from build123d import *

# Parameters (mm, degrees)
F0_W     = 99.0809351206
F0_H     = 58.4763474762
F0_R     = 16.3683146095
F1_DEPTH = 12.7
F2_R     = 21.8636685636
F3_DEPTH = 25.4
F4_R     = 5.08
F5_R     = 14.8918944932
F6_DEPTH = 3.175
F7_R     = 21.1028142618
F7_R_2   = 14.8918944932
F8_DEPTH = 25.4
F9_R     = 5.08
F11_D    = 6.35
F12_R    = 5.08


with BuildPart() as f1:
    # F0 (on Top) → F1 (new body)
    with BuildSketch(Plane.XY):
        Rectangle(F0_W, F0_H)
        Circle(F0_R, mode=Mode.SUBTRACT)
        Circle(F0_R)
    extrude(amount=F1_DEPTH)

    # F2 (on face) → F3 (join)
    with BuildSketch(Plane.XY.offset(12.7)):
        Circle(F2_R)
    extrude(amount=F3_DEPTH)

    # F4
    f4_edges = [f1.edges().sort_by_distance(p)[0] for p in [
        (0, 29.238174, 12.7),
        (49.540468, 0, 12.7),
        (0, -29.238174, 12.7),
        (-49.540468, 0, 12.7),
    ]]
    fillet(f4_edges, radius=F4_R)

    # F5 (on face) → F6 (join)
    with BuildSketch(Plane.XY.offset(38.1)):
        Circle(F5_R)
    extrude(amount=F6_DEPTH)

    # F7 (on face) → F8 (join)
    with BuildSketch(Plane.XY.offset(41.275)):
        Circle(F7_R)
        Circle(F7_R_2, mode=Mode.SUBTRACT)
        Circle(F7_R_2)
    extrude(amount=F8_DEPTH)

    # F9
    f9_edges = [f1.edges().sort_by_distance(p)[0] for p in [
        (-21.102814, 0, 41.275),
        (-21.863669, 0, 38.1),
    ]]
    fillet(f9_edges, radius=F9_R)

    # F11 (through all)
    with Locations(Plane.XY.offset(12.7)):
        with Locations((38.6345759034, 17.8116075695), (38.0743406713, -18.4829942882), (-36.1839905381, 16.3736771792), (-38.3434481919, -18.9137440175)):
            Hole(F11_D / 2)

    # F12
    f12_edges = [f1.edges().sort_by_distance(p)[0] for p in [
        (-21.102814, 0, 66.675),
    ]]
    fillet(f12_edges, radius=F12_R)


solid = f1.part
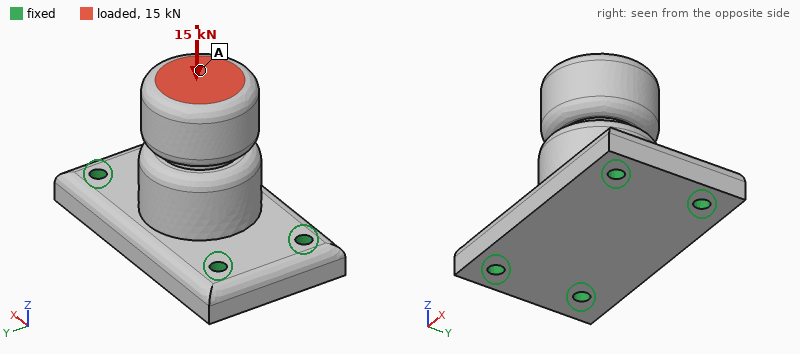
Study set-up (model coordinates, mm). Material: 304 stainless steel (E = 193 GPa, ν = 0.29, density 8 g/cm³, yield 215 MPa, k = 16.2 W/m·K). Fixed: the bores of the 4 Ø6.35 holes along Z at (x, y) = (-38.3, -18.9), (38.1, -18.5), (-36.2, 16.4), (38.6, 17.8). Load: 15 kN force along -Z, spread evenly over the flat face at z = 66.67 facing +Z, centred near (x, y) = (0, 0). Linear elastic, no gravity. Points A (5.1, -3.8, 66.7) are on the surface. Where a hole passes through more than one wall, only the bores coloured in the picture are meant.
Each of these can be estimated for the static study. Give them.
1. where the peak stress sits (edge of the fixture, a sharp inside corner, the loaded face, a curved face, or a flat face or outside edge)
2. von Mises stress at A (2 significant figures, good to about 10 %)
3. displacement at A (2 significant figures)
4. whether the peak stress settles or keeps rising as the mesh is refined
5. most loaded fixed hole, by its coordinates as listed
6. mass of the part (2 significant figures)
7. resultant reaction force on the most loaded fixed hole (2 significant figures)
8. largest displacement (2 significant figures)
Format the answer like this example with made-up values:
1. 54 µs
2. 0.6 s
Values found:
1. edge of the fixture
2. 12 MPa
3. 16 µm
4. keeps rising
5. (-36.2, 16.4)
6. 1.2 kg
7. 4.5 kN
8. 16 µm
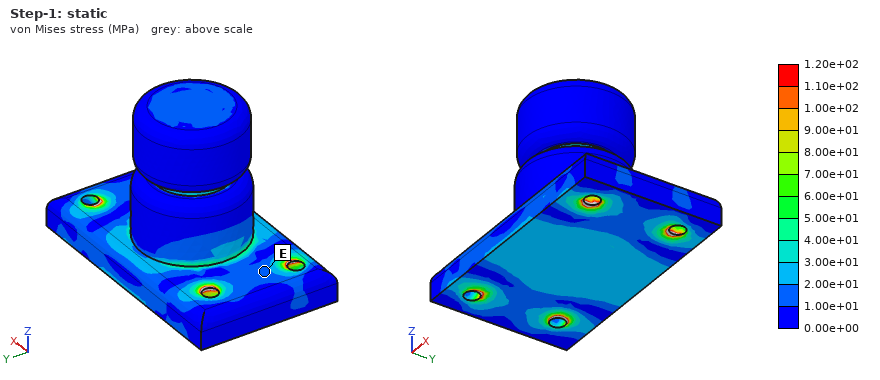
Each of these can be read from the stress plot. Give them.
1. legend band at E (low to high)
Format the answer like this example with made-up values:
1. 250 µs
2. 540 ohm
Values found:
1. 1.00e+01 to 2.00e+01 MPa
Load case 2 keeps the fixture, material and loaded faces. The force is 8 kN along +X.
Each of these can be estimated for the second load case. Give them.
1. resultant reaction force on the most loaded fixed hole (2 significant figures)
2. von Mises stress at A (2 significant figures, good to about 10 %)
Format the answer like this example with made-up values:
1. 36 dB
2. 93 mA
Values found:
1. 5.0 kN
2. 18 MPa
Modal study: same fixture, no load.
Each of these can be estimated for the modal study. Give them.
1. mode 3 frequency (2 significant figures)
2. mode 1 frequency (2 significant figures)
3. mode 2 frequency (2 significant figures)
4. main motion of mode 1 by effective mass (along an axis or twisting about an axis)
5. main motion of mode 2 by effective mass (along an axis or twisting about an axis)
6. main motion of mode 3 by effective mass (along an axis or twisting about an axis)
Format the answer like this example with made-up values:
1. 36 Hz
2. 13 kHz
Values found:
1. 6100 Hz
2. 3200 Hz
3. 4600 Hz
4. along Y
5. along X
6. along Z
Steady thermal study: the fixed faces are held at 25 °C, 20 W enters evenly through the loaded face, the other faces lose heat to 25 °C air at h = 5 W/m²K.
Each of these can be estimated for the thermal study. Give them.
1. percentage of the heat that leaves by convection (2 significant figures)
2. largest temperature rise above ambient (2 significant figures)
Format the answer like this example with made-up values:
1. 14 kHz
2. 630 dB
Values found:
1. 13 %
2. 80 K
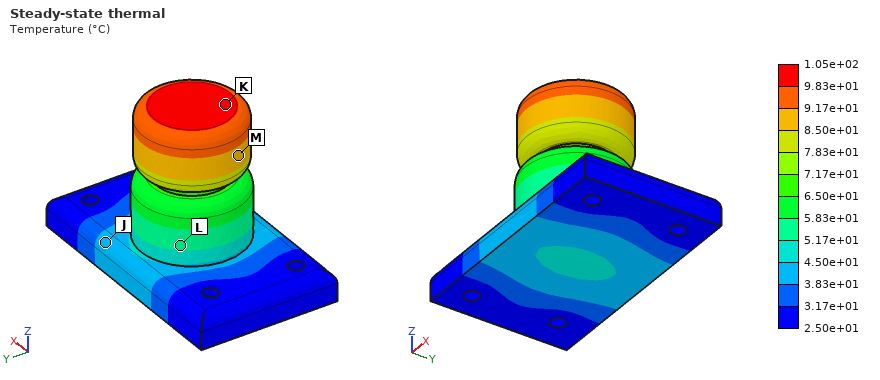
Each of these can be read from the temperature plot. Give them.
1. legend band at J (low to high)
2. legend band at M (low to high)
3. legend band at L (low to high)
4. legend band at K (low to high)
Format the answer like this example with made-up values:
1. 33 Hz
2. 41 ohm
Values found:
1. 3.83e+01 to 4.50e+01 °C
2. 8.50e+01 to 9.17e+01 °C
3. 5.17e+01 to 5.83e+01 °C
4. 9.83e+01 to 1.05e+02 °C
